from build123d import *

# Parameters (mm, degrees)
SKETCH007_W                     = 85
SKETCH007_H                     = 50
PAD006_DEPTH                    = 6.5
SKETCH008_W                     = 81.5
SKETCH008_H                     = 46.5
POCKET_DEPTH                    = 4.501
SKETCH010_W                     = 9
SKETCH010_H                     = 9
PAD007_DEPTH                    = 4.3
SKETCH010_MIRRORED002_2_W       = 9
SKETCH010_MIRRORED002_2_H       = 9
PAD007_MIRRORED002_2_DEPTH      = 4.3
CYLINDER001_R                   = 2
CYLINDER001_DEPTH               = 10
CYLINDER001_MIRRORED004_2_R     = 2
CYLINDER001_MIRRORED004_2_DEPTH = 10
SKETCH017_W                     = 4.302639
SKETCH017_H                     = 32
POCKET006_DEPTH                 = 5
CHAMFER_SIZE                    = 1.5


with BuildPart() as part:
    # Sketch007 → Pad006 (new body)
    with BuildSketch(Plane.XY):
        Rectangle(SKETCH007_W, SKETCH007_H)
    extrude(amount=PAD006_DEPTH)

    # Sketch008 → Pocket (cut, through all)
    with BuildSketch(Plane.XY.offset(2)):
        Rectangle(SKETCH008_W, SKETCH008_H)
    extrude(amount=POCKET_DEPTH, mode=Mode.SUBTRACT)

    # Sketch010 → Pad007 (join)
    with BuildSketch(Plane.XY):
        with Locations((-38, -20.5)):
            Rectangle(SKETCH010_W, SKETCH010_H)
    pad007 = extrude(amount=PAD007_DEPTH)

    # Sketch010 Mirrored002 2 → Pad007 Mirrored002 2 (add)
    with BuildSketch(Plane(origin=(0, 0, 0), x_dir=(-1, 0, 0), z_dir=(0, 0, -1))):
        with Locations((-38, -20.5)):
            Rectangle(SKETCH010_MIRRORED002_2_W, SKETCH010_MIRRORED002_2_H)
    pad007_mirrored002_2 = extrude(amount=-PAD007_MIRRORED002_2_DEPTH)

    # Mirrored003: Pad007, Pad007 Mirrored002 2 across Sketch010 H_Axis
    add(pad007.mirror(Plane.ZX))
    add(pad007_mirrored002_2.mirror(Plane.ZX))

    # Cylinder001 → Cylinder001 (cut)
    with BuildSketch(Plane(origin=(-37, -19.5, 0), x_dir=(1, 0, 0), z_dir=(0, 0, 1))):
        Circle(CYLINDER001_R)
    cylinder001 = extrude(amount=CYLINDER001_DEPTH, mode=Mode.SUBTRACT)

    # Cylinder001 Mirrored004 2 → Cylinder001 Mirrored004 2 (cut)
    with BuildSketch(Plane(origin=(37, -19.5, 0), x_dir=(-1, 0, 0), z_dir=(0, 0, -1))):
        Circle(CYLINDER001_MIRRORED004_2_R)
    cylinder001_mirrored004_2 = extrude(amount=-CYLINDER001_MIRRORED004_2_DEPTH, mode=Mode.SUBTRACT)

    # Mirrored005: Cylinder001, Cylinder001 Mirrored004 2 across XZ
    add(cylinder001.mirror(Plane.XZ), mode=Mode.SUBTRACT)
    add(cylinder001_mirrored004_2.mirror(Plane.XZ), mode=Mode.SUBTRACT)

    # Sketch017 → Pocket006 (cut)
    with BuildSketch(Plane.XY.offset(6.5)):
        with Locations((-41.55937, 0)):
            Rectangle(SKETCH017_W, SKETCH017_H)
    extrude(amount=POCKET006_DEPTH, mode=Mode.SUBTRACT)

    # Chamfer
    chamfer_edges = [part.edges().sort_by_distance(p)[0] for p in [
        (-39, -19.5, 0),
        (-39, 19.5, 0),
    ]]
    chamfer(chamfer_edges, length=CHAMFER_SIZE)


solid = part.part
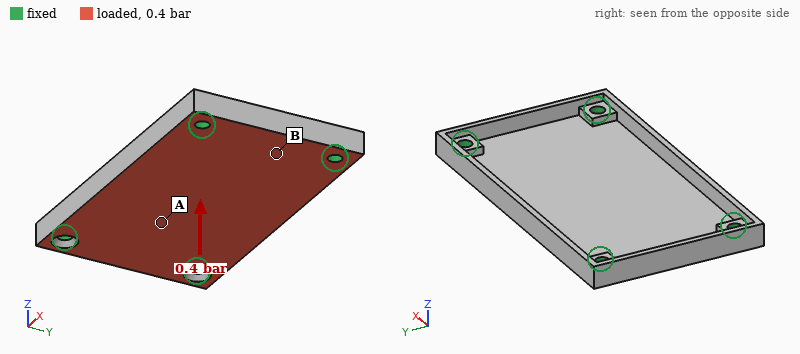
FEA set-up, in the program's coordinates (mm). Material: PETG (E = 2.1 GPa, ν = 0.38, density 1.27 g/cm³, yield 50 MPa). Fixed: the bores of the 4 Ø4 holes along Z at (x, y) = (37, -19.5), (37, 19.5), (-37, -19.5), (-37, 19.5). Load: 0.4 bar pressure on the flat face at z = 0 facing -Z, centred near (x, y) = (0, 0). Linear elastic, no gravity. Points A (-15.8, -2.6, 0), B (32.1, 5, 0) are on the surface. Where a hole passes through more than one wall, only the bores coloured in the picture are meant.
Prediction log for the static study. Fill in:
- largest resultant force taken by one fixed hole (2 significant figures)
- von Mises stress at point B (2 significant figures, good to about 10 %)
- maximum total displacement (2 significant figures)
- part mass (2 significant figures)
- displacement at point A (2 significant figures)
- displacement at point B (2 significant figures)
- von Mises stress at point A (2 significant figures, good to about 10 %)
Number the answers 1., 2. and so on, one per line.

1. 50 N
2. 4.1 MPa
3. 1.1 mm
4. 14 g
5. 0.82 mm
6. 0.22 mm
7. 6.8 MPa
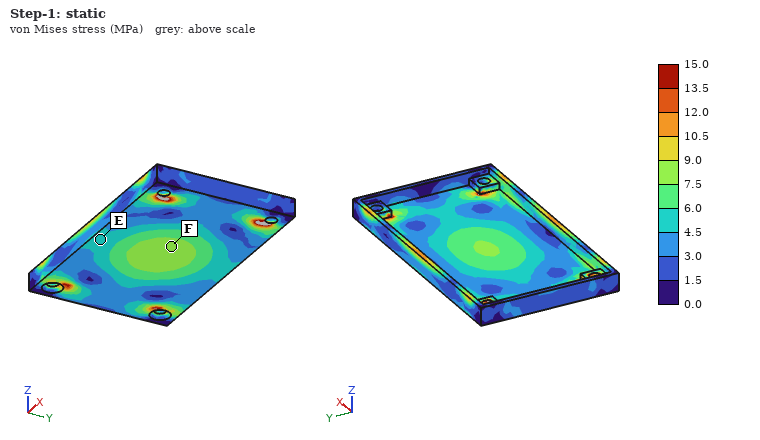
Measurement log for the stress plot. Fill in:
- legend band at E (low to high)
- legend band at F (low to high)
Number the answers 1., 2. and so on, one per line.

1. 4.5 to 6.0 MPa
2. 7.5 to 9.0 MPa
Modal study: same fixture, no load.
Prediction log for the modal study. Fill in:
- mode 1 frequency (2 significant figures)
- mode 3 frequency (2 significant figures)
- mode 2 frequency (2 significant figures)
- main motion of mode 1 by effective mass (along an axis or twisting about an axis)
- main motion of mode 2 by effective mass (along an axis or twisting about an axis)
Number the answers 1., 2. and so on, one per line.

1. 740 Hz
2. 1600 Hz
3. 1200 Hz
4. along Z
5. twisting about X
